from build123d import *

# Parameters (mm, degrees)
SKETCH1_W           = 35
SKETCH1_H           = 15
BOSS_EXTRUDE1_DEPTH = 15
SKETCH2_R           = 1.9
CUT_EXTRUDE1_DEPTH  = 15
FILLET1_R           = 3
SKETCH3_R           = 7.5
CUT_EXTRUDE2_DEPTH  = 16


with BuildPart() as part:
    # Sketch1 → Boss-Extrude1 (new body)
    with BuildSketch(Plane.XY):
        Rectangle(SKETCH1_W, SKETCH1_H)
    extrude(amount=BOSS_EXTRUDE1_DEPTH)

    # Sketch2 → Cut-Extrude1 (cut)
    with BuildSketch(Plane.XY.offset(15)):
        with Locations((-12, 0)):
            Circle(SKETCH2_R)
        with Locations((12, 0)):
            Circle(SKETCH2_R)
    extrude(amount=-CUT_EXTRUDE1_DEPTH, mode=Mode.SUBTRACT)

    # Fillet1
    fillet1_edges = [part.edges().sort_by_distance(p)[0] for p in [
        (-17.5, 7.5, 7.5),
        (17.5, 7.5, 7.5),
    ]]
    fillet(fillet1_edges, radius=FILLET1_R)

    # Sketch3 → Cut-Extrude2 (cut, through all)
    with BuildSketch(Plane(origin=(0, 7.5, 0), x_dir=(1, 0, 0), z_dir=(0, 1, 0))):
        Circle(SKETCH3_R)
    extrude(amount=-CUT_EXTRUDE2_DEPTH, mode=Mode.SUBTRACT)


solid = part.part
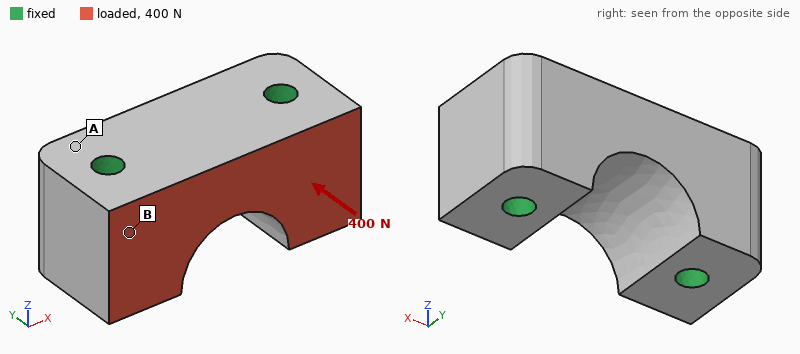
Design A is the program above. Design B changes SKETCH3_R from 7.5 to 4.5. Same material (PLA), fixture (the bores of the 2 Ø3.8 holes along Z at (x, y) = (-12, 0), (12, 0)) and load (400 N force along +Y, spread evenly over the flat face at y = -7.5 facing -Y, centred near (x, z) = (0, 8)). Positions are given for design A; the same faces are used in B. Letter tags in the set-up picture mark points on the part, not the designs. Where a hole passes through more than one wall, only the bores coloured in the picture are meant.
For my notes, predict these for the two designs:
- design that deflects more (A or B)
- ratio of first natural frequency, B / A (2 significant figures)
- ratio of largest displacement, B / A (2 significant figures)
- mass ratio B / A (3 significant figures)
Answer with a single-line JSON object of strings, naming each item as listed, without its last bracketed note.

{"design that deflects more": "A", "ratio of first natural frequency, B / A": "0.98", "ratio of largest displacement, B / A": "0.91", "mass ratio B / A": "1.14"}
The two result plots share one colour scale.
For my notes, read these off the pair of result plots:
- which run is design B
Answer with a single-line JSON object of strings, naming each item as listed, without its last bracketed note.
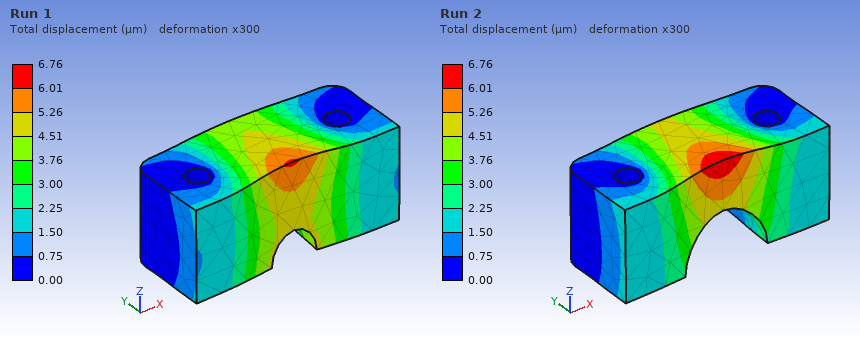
{"which run is design B": "Run 1"}
